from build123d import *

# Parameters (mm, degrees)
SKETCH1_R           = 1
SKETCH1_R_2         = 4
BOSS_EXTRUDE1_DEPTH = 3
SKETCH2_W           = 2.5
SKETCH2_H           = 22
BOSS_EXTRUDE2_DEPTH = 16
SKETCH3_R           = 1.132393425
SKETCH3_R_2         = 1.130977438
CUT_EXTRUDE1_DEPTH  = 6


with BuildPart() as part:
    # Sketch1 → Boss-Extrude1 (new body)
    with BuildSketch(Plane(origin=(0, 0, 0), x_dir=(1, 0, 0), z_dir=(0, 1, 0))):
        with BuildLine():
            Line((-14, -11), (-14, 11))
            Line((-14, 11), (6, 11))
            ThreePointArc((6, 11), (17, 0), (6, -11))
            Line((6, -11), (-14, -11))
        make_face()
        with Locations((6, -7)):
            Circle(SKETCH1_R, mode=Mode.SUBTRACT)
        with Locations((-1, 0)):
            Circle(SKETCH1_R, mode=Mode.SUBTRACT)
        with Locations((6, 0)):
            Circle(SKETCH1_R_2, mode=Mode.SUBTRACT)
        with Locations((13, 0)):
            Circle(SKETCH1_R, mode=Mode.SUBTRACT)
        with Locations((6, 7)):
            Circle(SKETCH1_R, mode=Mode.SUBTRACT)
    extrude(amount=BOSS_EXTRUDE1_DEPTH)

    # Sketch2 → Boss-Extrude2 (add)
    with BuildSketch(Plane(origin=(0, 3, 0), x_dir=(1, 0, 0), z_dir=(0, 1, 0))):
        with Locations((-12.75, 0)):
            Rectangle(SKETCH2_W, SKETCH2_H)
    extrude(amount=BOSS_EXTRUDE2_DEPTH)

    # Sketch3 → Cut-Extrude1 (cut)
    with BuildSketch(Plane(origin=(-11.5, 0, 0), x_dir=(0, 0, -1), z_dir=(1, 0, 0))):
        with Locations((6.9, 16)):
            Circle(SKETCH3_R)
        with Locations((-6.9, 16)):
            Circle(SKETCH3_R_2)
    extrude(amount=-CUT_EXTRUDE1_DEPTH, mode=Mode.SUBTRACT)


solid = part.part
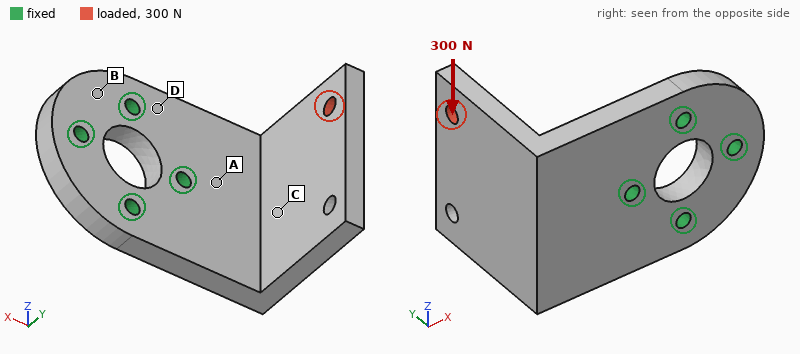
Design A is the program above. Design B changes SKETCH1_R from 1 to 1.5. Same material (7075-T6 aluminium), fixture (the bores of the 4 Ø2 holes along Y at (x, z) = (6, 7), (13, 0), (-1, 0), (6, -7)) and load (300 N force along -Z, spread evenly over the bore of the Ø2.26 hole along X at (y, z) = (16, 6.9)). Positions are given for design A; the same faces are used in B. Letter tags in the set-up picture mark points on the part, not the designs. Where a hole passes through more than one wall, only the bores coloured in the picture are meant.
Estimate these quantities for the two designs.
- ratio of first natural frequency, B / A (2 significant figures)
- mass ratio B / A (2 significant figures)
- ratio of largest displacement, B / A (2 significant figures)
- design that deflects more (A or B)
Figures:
1.0
0.98
0.91
A
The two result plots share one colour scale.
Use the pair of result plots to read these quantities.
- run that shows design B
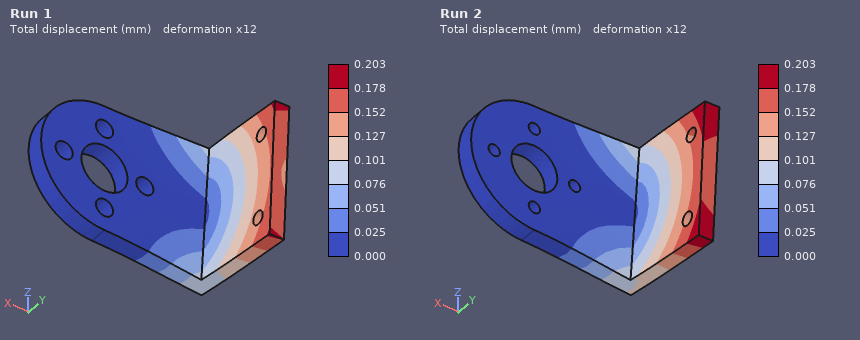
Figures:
Run 1
